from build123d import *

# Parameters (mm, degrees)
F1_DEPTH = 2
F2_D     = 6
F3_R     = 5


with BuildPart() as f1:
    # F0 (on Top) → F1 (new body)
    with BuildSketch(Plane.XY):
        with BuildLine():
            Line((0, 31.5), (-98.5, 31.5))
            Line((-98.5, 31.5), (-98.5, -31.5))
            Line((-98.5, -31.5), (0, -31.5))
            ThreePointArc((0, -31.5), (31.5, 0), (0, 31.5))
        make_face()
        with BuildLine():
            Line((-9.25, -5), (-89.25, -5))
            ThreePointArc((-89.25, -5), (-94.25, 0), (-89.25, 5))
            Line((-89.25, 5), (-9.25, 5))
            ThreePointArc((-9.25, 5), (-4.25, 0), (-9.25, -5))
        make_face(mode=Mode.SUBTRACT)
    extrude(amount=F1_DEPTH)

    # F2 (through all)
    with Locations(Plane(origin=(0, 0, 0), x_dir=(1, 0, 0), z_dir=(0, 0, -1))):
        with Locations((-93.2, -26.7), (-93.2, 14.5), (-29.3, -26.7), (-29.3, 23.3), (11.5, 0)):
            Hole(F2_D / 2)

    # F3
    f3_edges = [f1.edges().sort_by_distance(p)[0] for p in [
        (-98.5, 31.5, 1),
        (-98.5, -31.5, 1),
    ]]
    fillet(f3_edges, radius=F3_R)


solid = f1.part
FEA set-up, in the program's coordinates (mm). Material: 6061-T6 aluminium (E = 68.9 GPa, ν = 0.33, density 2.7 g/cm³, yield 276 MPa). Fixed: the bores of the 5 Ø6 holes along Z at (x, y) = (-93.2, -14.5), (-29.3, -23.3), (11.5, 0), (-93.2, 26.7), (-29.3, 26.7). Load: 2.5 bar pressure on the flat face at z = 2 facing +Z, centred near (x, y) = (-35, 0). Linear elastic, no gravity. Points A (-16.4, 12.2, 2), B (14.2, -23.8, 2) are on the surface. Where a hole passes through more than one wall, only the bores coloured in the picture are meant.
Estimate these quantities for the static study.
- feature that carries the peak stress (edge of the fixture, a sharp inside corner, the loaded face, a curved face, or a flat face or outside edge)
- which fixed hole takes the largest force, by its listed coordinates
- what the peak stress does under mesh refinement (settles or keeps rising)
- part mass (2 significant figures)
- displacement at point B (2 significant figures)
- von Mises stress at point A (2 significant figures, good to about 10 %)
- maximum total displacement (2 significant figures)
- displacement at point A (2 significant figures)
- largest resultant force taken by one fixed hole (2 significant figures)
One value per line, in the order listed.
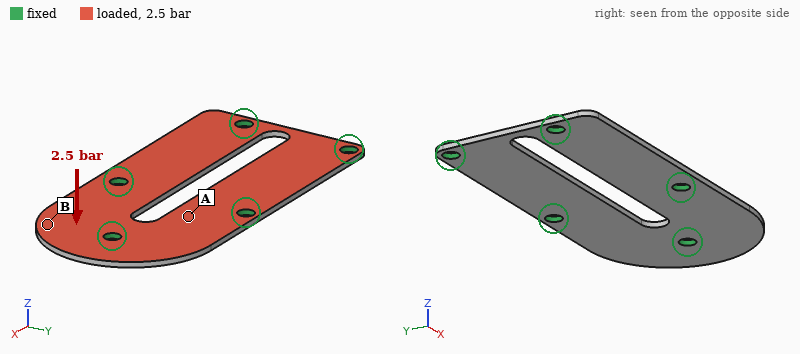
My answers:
edge of the fixture
(11.5, 0)
keeps rising
36 g
0.17 mm
45 MPa
0.40 mm
0.060 mm
460 N
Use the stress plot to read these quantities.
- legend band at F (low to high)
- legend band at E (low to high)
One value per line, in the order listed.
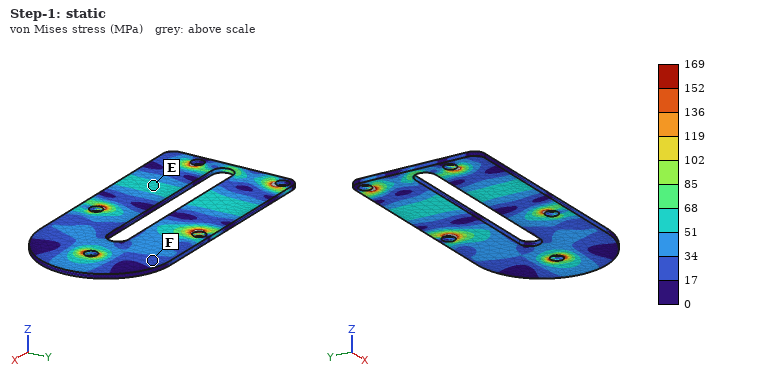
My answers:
17 to 34 MPa
51 to 68 MPa
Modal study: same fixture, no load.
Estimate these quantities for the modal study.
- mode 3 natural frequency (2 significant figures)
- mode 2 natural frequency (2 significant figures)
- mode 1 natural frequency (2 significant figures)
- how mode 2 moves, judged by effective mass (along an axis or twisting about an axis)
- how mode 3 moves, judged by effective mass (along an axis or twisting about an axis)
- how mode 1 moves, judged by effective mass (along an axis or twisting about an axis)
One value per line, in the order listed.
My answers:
2700 Hz
2600 Hz
2200 Hz
along Z
twisting about X
along Z
